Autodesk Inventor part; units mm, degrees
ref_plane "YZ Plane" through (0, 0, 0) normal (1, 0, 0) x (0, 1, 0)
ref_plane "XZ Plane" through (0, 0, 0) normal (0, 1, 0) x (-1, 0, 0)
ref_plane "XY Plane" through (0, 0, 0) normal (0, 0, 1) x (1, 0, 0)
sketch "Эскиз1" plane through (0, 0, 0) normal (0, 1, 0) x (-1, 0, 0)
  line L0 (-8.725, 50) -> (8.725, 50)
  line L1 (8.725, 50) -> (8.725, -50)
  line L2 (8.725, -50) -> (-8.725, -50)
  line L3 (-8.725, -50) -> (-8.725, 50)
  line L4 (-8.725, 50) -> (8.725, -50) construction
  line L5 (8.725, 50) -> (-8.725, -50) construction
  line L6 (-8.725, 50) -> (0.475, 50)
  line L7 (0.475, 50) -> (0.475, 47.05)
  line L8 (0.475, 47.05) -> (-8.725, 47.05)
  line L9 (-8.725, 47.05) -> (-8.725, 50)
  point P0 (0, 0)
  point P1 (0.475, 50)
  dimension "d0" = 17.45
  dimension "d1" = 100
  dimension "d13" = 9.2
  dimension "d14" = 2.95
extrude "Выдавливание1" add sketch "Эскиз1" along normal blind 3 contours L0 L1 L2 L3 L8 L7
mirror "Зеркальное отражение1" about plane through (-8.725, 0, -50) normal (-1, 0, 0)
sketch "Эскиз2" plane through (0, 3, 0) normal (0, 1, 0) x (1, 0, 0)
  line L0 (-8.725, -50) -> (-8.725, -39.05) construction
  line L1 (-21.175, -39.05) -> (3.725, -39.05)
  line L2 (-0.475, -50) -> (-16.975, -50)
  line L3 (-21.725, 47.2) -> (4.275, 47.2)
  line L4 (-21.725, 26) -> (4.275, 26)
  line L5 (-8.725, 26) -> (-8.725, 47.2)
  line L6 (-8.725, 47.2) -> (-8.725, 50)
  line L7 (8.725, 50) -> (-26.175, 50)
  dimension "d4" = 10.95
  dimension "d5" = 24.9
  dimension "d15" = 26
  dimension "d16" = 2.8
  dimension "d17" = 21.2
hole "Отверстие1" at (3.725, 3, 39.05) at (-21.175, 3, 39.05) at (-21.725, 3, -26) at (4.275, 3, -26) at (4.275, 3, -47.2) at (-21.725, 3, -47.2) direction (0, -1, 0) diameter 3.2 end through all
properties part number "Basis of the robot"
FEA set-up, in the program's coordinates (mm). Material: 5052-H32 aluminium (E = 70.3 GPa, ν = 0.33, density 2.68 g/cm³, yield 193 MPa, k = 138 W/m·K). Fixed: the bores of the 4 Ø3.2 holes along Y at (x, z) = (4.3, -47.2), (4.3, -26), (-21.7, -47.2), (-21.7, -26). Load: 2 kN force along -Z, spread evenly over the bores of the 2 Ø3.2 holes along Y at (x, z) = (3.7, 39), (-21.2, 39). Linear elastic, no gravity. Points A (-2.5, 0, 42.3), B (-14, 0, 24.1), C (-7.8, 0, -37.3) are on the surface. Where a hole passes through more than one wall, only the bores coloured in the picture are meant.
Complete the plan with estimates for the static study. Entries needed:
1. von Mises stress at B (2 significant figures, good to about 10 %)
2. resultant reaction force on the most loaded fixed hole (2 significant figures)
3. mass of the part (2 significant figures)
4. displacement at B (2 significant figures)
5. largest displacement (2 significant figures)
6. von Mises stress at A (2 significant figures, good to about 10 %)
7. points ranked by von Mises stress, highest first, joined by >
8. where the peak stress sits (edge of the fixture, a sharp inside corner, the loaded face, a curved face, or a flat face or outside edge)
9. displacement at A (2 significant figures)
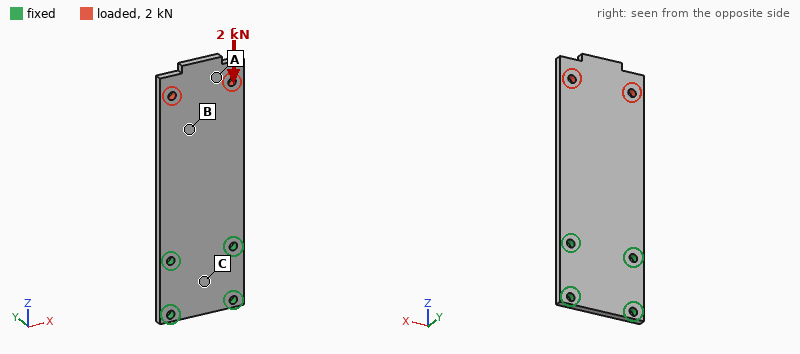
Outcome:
17 MPa
860 N
27 g
14 µm
21 µm
11 MPa
B > A > C
the loaded face
18 µm
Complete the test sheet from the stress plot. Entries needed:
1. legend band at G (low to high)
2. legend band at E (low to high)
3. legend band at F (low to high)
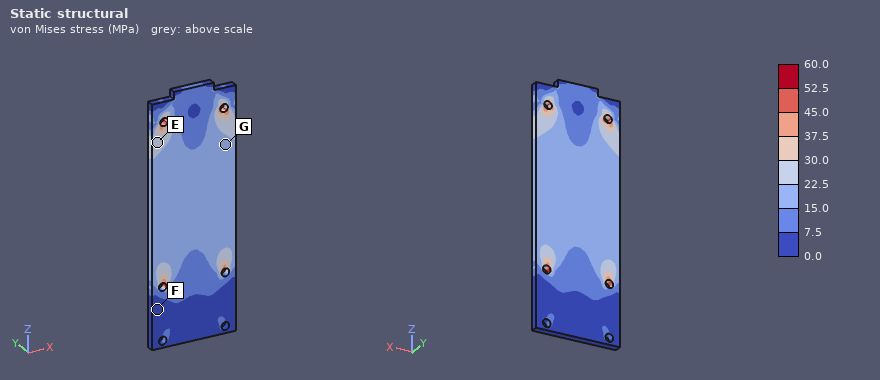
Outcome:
15.0 to 22.5 MPa
22.5 to 30.0 MPa
0.0 to 7.5 MPa
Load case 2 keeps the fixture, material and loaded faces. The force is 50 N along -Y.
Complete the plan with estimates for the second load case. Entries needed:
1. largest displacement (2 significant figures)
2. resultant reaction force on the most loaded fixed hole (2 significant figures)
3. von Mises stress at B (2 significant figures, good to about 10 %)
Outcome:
1.0 mm
47 N
14 MPa
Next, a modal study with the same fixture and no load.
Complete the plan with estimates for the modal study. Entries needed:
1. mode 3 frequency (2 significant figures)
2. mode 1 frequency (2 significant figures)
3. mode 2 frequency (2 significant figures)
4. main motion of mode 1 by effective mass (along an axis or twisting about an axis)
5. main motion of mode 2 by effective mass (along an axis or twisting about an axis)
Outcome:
2800 Hz
450 Hz
2100 Hz
along Y
twisting about Z
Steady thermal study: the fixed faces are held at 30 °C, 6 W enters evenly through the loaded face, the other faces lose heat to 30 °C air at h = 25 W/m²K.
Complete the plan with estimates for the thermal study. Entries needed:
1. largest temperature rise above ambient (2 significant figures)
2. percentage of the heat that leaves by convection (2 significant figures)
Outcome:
23 K
29 %
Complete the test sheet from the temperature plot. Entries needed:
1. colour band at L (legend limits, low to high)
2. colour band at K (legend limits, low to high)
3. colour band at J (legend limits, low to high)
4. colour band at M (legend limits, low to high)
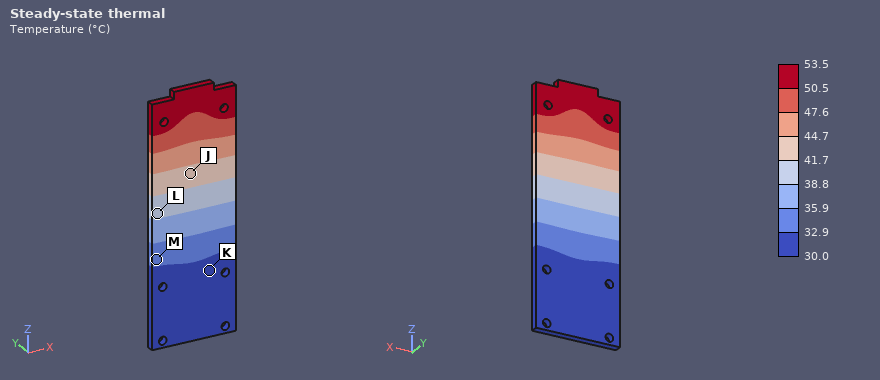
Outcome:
38.8 to 41.7 °C
30.0 to 32.9 °C
41.7 to 44.7 °C
32.9 to 35.9 °C
